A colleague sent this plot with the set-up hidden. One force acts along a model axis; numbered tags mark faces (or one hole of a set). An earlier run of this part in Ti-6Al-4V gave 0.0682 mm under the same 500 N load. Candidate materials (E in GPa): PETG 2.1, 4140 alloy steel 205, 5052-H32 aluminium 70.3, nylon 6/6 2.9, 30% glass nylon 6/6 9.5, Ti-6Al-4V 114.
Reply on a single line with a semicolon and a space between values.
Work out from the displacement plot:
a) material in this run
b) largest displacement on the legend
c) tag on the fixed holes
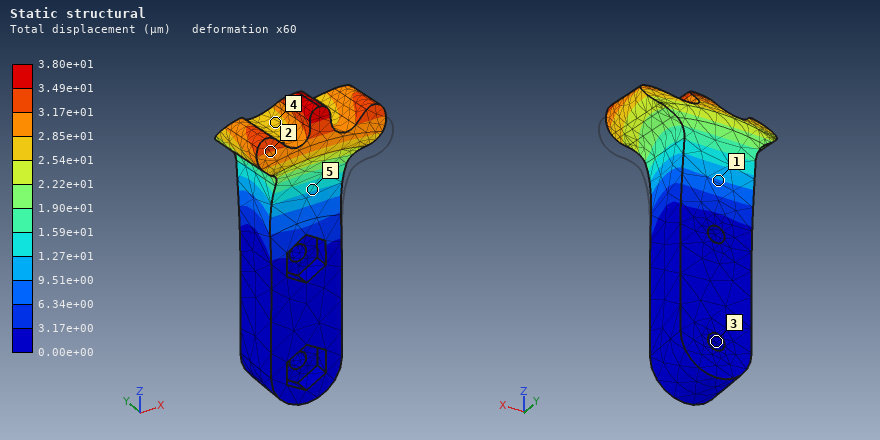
4140 alloy steel; 3.80e+01 µm; 3
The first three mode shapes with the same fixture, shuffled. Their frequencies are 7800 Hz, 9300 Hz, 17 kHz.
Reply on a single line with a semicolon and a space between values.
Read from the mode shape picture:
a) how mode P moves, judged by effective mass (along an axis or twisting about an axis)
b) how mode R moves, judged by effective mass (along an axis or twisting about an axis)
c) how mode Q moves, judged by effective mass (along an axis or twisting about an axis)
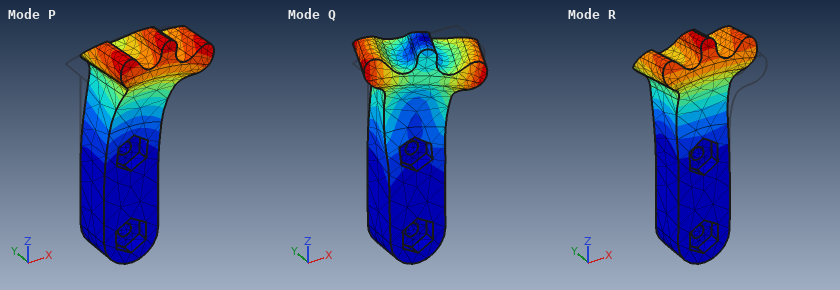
along X; along Y; twisting about Z
